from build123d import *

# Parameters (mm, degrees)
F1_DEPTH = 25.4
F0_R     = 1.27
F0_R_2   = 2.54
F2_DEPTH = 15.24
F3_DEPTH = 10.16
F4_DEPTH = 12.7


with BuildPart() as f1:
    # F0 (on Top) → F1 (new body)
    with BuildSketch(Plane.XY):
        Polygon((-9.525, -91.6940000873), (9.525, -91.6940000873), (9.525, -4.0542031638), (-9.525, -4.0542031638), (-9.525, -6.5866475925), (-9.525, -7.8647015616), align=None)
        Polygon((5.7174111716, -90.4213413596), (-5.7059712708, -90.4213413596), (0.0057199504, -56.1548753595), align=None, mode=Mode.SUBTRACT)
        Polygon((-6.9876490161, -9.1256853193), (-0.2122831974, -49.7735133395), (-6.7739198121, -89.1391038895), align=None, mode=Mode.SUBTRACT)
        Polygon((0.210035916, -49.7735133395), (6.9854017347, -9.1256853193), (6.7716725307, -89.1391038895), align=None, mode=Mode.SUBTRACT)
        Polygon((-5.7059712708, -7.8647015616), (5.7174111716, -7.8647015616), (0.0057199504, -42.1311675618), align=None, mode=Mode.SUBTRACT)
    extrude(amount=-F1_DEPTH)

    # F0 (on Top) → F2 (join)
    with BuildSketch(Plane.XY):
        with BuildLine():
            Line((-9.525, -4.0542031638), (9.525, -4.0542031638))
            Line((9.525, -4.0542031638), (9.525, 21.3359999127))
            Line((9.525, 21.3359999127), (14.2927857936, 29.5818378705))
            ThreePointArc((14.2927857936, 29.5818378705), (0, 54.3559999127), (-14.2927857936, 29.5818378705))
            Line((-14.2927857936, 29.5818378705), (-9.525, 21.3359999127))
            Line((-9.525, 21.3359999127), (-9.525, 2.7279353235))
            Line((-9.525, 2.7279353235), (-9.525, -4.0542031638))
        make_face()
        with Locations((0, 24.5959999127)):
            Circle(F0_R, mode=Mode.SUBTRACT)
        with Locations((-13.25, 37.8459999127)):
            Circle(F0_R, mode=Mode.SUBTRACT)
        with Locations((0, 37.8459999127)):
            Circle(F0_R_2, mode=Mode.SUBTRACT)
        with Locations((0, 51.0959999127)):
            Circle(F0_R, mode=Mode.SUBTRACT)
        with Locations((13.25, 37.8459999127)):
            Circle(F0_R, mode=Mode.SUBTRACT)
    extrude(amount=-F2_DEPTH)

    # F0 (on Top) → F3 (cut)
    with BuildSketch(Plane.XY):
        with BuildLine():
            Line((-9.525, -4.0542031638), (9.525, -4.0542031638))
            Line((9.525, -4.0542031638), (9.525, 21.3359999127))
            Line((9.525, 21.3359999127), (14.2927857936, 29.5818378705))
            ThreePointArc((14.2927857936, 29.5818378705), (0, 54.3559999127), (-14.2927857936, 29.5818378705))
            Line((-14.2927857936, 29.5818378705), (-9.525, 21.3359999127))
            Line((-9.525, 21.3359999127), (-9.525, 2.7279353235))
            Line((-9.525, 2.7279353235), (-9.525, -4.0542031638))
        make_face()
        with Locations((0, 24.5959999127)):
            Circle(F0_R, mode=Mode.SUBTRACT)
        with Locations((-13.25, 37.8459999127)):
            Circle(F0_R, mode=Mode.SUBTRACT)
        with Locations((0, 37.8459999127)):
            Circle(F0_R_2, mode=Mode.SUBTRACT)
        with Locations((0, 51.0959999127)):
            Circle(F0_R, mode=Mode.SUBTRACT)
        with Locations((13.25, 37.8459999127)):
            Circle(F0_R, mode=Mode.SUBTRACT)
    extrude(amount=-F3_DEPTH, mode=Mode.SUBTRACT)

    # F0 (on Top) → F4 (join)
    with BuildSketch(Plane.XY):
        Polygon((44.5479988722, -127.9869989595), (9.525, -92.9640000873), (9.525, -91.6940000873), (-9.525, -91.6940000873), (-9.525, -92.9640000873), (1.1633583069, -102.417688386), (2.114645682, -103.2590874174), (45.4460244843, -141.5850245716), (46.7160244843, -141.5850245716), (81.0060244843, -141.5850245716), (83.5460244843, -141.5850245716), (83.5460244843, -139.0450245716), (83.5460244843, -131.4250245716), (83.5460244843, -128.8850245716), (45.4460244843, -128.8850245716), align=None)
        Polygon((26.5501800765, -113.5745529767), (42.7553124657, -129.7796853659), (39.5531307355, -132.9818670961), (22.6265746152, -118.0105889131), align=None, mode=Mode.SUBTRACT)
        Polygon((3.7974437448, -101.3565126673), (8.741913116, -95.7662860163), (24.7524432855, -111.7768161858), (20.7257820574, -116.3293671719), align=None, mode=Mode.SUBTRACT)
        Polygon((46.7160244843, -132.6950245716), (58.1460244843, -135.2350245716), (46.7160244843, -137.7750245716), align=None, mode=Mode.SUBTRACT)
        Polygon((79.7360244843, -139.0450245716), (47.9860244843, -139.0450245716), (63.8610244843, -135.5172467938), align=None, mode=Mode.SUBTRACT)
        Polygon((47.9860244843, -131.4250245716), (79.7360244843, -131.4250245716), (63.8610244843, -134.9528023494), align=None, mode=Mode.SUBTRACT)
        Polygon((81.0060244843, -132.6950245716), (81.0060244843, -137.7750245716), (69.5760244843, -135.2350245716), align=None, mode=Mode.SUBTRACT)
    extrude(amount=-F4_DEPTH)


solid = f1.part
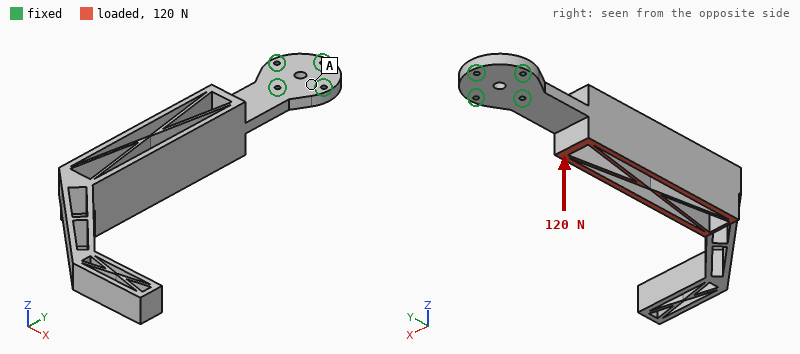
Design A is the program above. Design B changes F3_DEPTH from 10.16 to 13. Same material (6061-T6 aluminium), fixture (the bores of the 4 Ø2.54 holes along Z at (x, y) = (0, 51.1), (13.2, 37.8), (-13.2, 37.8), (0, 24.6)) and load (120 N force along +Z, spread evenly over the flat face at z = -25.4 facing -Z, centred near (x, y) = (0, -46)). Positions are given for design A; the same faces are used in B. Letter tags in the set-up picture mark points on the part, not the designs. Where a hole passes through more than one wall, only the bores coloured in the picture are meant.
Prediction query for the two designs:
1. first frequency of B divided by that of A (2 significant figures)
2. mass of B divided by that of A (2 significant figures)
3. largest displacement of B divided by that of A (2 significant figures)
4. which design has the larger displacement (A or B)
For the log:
0.32
0.89
11
B
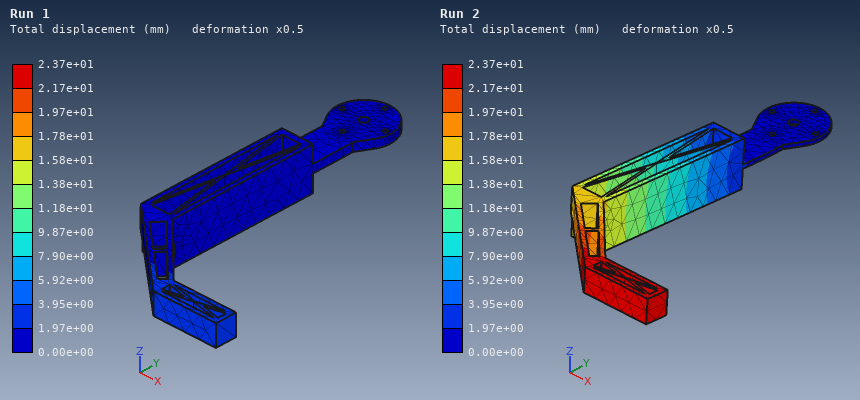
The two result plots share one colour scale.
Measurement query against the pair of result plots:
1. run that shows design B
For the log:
Run 2
